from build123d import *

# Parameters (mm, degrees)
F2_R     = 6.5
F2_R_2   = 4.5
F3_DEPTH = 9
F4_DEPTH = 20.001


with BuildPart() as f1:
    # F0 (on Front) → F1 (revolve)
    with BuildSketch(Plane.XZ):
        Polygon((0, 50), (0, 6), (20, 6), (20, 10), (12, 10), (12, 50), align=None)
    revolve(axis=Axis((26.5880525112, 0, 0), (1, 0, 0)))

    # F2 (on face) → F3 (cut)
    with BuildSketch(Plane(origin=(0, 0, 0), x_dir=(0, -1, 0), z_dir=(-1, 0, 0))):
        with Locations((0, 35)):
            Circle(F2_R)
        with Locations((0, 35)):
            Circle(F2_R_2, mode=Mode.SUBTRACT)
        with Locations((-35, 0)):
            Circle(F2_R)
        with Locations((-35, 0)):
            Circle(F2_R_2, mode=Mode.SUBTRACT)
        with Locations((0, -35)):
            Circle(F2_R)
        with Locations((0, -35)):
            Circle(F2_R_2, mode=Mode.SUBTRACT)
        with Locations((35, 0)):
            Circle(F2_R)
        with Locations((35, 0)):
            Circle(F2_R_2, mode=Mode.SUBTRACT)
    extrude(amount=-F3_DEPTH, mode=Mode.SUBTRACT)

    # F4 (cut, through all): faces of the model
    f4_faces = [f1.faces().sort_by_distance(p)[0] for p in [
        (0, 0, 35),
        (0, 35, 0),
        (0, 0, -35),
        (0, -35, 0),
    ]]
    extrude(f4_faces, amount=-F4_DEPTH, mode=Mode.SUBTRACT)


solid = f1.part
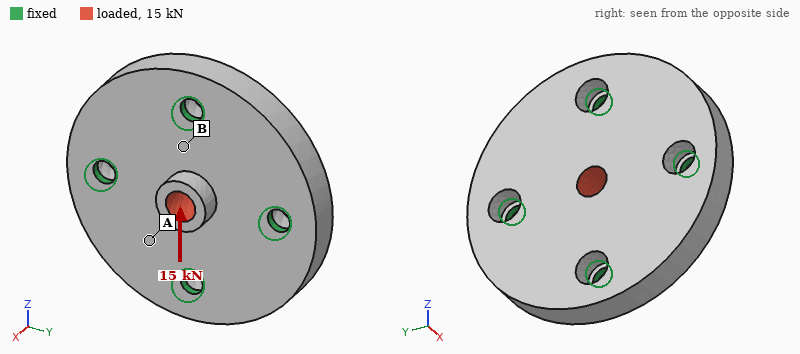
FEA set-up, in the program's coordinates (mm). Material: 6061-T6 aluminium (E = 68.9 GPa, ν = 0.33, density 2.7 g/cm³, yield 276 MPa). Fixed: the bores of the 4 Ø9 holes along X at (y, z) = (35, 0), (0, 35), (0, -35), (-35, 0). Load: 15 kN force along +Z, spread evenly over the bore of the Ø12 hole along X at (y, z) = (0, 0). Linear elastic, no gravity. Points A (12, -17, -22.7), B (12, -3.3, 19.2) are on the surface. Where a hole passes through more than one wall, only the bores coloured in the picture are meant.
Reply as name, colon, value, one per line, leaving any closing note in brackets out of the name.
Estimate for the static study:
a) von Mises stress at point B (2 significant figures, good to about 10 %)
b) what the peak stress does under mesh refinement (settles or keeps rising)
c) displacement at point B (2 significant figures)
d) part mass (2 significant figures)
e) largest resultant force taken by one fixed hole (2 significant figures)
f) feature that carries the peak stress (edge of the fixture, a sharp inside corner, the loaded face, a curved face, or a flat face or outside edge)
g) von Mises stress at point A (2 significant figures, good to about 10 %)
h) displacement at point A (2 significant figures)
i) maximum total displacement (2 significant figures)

von Mises stress at point B: 39 MPa
what the peak stress does under mesh refinement: keeps rising
displacement at point B: 9.3 µm
part mass: 240 g
largest resultant force taken by one fixed hole: 4.2 kN
feature that carries the peak stress: edge of the fixture
von Mises stress at point A: 12 MPa
displacement at point A: 6.2 µm
maximum total displacement: 34 µm
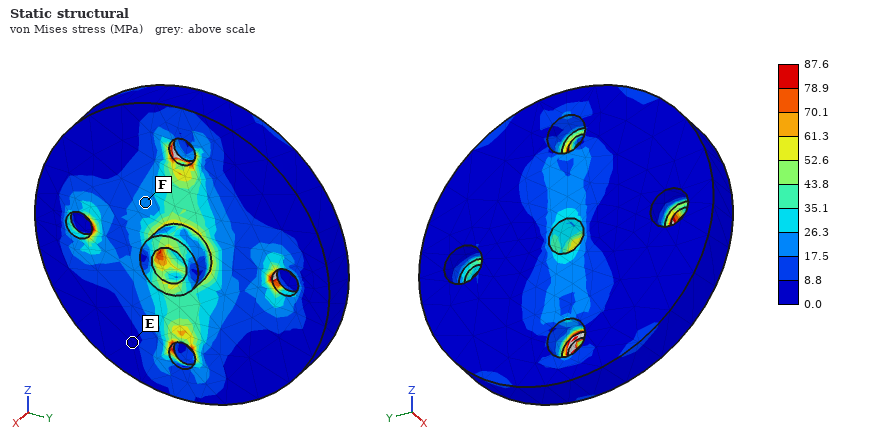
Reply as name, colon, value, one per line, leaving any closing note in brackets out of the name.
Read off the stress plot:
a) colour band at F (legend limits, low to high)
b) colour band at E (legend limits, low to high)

colour band at F: 17.5 to 26.3 MPa
colour band at E: 0.0 to 8.8 MPa
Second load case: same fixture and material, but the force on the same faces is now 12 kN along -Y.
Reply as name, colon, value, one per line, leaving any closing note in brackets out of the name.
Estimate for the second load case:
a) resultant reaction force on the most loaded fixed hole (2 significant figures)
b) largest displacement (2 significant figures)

resultant reaction force on the most loaded fixed hole: 3.4 kN
largest displacement: 27 µm
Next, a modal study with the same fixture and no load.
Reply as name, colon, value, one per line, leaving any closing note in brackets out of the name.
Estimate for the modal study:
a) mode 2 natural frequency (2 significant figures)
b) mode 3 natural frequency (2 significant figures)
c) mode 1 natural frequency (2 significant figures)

mode 2 natural frequency: 9300 Hz
mode 3 natural frequency: 9300 Hz
mode 1 natural frequency: 8400 Hz
